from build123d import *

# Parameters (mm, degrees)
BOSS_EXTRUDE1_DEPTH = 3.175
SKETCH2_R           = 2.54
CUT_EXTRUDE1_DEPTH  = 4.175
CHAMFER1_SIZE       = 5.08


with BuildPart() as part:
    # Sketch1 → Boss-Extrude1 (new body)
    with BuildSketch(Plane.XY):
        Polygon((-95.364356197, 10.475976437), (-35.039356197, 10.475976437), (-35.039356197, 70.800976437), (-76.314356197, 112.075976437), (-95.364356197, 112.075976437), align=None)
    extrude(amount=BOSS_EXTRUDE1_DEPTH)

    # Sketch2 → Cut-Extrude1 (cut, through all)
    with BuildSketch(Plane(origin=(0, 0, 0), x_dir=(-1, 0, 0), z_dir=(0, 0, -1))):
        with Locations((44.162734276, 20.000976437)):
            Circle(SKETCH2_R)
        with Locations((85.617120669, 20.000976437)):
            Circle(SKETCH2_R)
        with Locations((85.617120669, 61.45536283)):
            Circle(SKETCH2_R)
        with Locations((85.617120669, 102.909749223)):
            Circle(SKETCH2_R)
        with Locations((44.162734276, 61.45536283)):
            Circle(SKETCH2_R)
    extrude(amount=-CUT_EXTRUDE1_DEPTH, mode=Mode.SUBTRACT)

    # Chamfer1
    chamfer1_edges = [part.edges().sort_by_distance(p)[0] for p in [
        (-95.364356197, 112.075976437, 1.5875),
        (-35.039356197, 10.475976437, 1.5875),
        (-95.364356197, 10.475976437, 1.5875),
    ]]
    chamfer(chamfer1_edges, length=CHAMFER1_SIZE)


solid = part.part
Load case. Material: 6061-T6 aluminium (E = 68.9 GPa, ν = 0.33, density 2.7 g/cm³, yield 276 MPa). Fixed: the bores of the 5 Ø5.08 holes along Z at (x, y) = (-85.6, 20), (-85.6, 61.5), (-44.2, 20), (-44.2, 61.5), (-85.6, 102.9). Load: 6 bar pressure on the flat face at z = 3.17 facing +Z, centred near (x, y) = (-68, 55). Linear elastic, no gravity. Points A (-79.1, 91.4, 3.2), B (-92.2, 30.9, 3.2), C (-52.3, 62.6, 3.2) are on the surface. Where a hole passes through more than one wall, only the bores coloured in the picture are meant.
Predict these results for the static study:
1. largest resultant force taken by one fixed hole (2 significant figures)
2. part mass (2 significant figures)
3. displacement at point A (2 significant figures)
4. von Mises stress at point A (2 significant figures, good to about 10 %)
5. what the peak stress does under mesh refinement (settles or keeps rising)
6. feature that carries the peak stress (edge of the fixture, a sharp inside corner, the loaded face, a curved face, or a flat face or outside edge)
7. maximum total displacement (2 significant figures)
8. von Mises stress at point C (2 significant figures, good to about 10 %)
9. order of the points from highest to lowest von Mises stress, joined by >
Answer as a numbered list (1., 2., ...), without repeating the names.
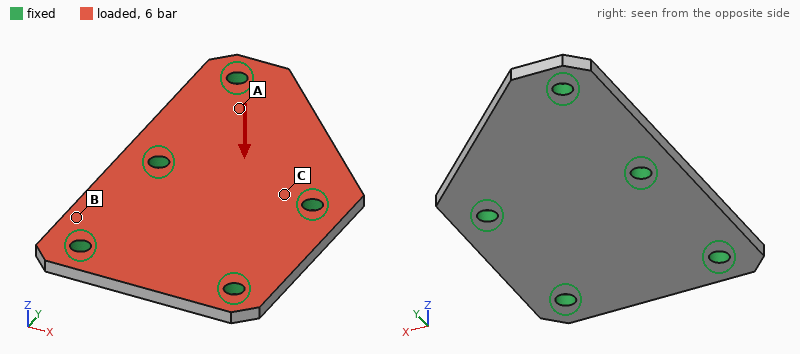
1. 760 N
2. 44 g
3. 0.032 mm
4. 26 MPa
5. keeps rising
6. edge of the fixture
7. 0.11 mm
8. 45 MPa
9. C > A > B
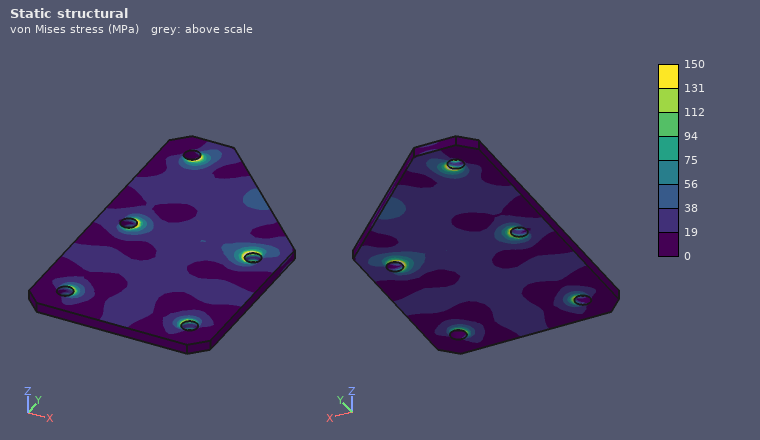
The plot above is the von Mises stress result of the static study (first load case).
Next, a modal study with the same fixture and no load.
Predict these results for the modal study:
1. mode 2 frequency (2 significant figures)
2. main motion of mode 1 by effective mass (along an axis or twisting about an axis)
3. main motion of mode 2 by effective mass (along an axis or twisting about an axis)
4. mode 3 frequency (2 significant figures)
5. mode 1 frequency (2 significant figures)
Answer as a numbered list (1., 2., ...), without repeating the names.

1. 7500 Hz
2. along Z
3. along Z
4. 10 kHz
5. 5300 Hz
